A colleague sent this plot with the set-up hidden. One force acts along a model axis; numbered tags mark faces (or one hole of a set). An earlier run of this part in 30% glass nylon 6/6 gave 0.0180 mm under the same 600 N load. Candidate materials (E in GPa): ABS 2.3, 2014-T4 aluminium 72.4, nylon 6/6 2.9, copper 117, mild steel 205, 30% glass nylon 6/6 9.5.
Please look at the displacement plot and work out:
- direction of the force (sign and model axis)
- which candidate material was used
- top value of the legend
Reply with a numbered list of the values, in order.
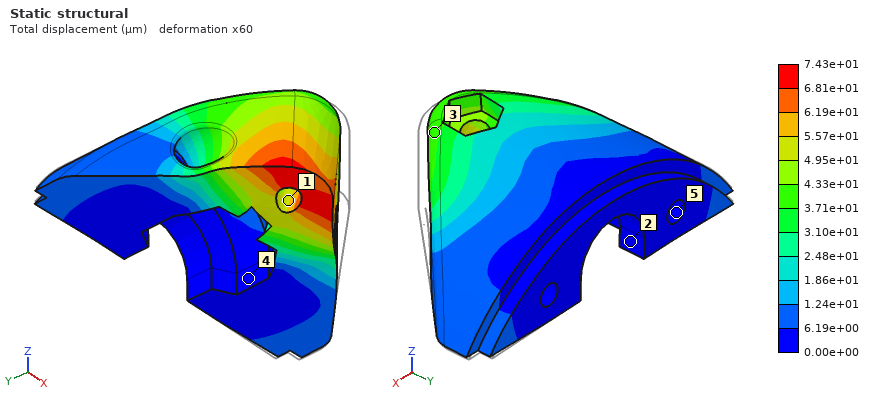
1. -X
2. ABS
3. 7.43e+01 µm
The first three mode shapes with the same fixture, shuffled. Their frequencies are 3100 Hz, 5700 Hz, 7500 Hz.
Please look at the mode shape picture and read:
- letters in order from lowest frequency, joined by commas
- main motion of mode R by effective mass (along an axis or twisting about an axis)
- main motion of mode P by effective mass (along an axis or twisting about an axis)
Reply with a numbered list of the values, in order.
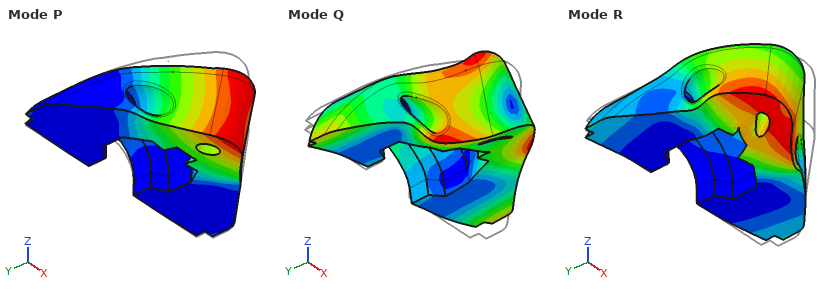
1. P, R, Q
2. along X
3. along Z
